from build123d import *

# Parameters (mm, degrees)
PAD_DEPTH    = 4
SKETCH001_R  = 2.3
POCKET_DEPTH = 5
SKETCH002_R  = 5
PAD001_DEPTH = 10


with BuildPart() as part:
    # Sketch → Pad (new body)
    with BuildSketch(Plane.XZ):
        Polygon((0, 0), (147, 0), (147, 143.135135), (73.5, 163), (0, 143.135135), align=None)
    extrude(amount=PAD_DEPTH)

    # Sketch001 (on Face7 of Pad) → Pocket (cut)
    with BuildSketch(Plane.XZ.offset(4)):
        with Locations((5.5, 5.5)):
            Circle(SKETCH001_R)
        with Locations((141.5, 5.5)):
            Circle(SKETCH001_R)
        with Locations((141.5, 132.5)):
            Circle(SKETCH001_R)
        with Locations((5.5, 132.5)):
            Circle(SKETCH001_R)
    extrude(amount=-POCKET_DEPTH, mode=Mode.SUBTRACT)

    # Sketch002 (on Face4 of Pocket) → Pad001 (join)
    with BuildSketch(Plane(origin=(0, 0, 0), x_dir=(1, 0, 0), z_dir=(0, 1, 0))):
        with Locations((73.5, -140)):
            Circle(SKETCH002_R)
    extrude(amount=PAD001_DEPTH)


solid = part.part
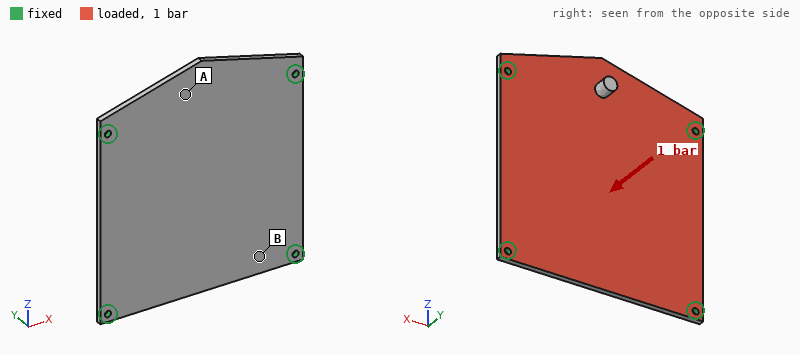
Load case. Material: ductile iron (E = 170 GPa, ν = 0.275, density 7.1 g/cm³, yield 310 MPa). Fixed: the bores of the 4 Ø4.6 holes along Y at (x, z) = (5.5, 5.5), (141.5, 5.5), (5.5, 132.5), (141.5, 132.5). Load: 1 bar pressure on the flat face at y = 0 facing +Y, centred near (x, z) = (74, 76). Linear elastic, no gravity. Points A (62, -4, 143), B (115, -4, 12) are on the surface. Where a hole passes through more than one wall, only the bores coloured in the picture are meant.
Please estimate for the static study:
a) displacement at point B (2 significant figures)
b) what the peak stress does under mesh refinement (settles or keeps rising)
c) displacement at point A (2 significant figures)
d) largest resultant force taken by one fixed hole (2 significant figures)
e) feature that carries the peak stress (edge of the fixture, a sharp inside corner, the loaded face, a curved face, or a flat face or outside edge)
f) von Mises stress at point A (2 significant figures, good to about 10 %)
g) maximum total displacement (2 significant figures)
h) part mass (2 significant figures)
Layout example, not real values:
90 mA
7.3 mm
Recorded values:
0.091 mm
keeps rising
0.14 mm
620 N
edge of the fixture
39 MPa
0.27 mm
640 g
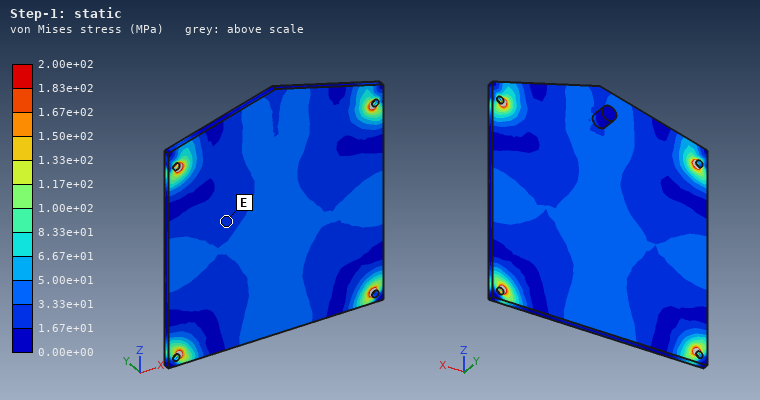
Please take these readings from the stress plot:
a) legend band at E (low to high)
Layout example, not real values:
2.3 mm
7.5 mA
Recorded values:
1.67e+01 to 3.33e+01 MPa
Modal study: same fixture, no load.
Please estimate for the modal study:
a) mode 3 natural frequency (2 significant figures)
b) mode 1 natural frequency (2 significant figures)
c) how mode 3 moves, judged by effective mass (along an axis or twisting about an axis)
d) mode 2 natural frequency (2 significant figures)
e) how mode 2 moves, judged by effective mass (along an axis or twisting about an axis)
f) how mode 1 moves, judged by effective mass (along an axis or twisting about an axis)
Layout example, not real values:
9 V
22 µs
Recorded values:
1300 Hz
690 Hz
twisting about Z
1000 Hz
twisting about X
along Y
